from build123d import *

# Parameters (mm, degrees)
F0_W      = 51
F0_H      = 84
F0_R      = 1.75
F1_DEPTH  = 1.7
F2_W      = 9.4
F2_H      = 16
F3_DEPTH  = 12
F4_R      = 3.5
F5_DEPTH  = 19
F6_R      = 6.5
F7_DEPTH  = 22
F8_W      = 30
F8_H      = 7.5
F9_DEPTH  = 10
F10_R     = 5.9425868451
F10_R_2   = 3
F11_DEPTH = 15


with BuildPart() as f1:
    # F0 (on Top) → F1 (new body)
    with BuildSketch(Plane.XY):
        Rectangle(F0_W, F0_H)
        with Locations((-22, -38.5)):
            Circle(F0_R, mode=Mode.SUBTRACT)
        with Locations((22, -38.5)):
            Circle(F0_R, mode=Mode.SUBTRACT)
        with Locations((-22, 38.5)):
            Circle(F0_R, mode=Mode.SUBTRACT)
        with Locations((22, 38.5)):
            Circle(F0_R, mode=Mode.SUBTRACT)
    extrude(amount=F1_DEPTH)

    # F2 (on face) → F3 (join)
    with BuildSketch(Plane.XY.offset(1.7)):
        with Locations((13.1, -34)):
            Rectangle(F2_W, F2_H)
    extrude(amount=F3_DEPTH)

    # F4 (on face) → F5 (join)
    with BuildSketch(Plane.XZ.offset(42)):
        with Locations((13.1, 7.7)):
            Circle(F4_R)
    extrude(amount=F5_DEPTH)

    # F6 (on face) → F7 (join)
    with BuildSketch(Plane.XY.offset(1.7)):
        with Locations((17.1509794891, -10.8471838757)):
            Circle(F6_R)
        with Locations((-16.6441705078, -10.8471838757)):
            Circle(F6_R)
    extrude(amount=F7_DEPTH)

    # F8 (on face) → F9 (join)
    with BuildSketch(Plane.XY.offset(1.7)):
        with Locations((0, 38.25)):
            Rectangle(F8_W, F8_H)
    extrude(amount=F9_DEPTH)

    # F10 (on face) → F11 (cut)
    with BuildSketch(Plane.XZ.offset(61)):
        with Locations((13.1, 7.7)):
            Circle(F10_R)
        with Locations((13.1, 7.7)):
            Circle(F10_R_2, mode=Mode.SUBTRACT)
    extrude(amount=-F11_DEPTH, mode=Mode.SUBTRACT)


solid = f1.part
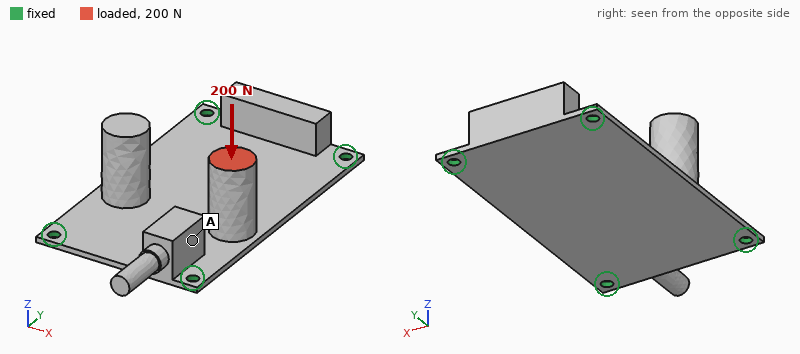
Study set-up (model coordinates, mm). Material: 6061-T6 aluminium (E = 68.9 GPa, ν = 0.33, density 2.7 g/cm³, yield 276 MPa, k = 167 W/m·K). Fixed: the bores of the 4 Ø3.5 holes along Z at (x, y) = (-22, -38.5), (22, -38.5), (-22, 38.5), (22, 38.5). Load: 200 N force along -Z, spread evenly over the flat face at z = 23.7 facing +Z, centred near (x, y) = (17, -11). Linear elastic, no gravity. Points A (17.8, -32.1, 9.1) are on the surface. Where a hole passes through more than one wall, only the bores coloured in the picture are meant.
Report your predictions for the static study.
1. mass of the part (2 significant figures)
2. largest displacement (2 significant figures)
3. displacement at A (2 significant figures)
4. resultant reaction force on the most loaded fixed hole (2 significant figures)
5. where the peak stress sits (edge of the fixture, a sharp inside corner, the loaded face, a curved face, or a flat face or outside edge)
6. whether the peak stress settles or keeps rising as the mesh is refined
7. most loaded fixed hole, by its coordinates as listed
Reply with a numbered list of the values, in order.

1. 48 g
2. 0.39 mm
3. 0.091 mm
4. 130 N
5. edge of the fixture
6. keeps rising
7. (22, -38.5)
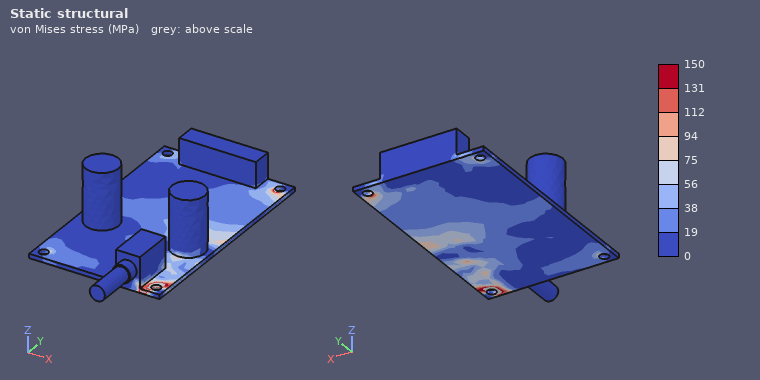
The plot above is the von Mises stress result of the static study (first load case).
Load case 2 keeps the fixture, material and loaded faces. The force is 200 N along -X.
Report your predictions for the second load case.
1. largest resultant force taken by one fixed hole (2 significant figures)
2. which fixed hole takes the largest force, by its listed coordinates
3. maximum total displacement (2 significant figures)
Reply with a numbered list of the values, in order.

1. 150 N
2. (22, -38.5)
3. 0.65 mm
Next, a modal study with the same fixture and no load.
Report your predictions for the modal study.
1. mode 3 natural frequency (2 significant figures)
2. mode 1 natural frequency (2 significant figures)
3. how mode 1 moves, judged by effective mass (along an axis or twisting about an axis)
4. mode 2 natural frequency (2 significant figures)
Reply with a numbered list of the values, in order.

1. 1500 Hz
2. 920 Hz
3. along Z
4. 1200 Hz
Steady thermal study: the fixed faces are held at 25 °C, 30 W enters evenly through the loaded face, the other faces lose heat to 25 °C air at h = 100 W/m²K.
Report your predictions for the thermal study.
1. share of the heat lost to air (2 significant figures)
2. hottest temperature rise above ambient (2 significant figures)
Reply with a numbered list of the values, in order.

1. 55 %
2. 66 K
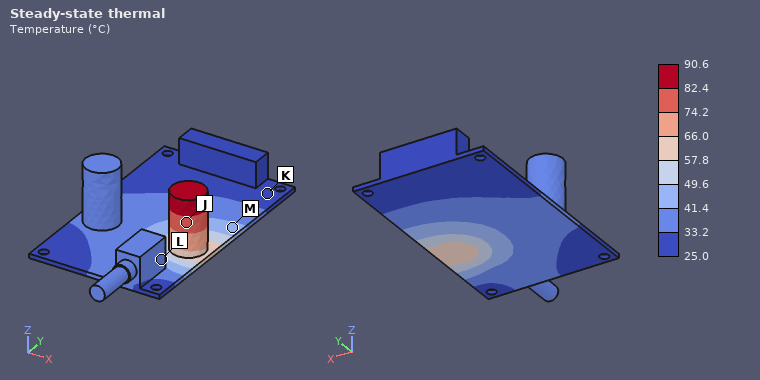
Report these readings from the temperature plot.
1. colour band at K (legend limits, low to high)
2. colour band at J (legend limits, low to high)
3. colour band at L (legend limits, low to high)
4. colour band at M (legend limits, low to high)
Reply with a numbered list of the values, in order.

1. 25.0 to 33.2 °C
2. 74.2 to 82.4 °C
3. 33.2 to 41.4 °C
4. 41.4 to 49.6 °C
